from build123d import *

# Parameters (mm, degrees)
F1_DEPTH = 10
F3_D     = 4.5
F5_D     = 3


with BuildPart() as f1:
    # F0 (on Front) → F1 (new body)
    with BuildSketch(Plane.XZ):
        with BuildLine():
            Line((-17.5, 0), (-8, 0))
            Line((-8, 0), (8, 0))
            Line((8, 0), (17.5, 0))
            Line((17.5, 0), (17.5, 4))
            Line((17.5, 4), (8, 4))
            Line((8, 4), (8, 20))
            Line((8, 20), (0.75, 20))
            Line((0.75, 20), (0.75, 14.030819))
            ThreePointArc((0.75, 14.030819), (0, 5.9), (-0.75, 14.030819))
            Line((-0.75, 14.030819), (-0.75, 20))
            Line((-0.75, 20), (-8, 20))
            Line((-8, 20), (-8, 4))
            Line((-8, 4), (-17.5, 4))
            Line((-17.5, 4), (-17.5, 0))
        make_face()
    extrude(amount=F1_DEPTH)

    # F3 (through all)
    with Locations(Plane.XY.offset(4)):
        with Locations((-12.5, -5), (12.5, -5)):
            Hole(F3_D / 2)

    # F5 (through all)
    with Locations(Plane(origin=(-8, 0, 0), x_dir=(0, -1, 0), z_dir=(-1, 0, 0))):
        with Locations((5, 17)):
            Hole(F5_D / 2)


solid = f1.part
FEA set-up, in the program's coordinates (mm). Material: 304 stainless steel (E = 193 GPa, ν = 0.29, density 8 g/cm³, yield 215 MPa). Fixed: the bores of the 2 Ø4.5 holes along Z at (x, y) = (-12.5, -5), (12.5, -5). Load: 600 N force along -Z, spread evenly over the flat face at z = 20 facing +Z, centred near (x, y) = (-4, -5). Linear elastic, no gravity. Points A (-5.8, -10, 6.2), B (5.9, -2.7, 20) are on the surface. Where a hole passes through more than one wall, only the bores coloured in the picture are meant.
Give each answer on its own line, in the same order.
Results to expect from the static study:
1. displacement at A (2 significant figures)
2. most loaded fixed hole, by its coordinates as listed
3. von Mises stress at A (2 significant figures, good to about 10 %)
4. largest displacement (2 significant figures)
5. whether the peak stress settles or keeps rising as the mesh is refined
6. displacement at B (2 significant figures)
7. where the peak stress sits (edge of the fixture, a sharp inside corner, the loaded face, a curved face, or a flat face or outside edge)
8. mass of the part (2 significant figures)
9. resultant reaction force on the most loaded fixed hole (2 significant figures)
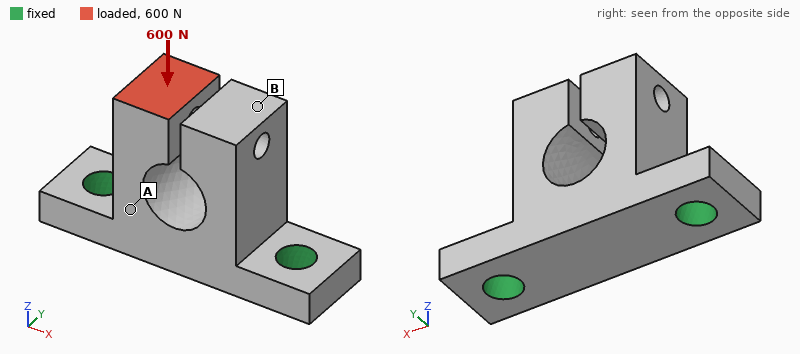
1.5 µm
(-12.5, -5)
18 MPa
9.9 µm
keeps rising
2.5 µm
edge of the fixture
25 g
470 N
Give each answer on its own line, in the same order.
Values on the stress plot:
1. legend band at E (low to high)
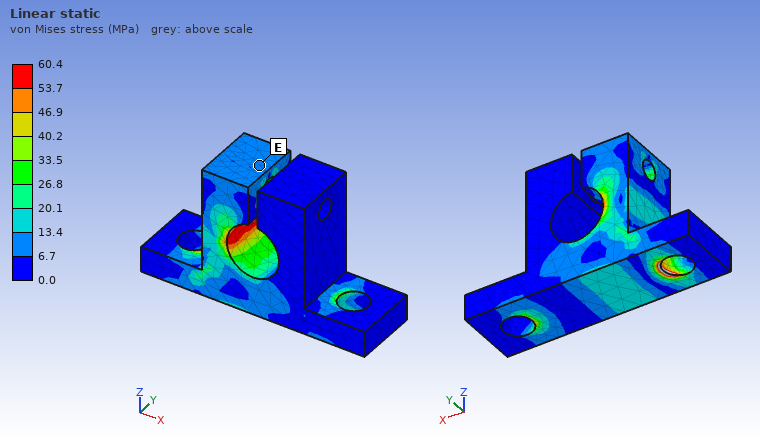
6.7 to 13.4 MPa
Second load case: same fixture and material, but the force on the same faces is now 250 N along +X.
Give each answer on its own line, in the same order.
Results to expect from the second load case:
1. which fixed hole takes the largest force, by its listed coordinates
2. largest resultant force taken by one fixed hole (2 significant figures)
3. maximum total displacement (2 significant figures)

(12.5, -5)
350 N
28 µm
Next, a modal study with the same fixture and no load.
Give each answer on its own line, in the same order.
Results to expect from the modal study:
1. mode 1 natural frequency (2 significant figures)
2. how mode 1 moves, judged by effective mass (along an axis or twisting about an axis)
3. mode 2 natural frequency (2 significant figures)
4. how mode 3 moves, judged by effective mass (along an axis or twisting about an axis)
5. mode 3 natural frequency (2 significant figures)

8500 Hz
along Y
10 kHz
along X
11 kHz
